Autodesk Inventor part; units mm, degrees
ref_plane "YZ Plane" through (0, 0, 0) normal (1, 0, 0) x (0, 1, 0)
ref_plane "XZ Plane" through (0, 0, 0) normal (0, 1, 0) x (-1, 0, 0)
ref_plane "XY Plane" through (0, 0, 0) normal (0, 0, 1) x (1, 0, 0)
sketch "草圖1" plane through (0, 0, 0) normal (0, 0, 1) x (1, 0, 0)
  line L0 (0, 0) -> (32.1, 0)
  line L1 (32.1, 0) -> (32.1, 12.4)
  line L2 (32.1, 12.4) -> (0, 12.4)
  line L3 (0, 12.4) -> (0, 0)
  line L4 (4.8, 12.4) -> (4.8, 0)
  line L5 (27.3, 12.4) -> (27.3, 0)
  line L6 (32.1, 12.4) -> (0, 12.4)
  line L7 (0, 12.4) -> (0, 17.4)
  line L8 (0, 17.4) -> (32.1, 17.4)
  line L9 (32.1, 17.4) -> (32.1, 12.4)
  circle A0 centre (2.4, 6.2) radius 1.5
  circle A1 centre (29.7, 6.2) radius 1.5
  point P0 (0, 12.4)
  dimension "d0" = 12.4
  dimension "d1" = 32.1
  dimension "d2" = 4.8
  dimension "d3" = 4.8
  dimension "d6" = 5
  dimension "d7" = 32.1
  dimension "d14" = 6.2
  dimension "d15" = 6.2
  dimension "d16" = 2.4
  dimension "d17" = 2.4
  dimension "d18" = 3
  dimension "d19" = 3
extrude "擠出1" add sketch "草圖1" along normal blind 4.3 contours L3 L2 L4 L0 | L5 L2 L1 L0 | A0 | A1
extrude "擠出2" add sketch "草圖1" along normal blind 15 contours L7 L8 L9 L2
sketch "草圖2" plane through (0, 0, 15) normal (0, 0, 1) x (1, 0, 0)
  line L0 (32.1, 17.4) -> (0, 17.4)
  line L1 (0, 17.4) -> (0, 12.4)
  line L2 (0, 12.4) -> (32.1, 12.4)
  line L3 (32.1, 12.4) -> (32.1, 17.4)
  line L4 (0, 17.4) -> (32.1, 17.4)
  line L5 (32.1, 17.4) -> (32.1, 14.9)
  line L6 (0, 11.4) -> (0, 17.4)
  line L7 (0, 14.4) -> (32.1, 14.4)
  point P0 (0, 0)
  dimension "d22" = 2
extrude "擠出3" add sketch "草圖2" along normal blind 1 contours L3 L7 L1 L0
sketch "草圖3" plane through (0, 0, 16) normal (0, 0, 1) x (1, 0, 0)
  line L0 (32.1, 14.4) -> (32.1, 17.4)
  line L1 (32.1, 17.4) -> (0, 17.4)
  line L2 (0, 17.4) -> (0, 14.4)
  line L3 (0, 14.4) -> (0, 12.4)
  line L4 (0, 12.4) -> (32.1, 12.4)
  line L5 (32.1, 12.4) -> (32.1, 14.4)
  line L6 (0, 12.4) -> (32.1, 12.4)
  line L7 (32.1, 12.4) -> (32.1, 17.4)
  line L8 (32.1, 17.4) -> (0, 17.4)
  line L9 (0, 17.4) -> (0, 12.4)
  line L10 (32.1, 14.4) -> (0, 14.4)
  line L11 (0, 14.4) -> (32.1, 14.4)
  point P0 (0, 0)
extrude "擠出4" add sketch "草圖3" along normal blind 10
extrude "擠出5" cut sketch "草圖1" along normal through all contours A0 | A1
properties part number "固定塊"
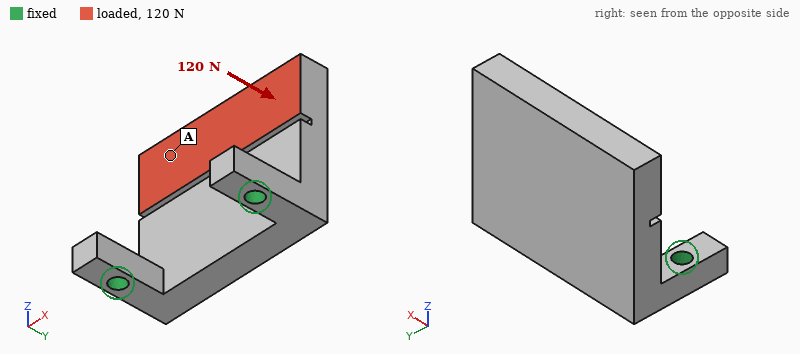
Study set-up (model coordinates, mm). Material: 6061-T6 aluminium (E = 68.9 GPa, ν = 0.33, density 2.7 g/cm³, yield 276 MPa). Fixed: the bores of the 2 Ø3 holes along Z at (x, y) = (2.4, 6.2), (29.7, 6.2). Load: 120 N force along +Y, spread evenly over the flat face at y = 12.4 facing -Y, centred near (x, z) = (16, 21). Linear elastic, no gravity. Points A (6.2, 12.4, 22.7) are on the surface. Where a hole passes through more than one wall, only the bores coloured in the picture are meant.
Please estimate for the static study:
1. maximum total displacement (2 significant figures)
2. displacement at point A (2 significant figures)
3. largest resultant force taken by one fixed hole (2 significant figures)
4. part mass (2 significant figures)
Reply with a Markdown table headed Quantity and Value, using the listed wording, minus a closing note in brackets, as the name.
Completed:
| Quantity | Value |
|---|---|
| maximum total displacement | 0.11 mm |
| displacement at point A | 0.091 mm |
| largest resultant force taken by one fixed hole | 63 N |
| part mass | 12 g |
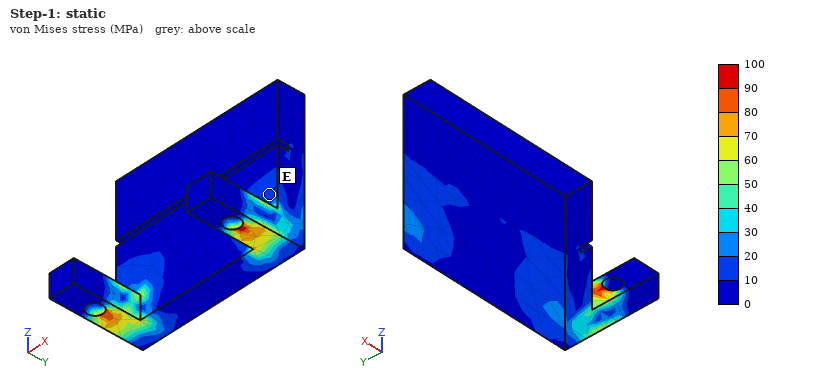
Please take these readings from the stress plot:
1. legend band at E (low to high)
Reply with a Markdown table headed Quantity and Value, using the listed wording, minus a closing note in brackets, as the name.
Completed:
| Quantity | Value |
|---|---|
| legend band at E | 10 to 20 MPa |
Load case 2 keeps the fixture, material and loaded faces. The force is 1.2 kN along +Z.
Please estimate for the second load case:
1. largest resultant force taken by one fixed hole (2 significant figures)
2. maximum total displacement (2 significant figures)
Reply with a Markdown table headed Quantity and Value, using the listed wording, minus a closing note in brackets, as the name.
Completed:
| Quantity | Value |
|---|---|
| largest resultant force taken by one fixed hole | 600 N |
| maximum total displacement | 51 µm |
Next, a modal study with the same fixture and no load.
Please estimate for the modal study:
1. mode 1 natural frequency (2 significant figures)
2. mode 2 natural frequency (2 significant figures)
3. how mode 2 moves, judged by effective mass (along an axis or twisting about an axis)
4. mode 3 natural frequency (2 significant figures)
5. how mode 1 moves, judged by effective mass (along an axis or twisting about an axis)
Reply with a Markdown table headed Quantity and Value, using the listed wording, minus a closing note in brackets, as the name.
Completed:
| Quantity | Value |
|---|---|
| mode 1 natural frequency | 2500 Hz |
| mode 2 natural frequency | 7300 Hz |
| how mode 2 moves, judged by effective mass | along X |
| mode 3 natural frequency | 11 kHz |
| how mode 1 moves, judged by effective mass | along Y |
